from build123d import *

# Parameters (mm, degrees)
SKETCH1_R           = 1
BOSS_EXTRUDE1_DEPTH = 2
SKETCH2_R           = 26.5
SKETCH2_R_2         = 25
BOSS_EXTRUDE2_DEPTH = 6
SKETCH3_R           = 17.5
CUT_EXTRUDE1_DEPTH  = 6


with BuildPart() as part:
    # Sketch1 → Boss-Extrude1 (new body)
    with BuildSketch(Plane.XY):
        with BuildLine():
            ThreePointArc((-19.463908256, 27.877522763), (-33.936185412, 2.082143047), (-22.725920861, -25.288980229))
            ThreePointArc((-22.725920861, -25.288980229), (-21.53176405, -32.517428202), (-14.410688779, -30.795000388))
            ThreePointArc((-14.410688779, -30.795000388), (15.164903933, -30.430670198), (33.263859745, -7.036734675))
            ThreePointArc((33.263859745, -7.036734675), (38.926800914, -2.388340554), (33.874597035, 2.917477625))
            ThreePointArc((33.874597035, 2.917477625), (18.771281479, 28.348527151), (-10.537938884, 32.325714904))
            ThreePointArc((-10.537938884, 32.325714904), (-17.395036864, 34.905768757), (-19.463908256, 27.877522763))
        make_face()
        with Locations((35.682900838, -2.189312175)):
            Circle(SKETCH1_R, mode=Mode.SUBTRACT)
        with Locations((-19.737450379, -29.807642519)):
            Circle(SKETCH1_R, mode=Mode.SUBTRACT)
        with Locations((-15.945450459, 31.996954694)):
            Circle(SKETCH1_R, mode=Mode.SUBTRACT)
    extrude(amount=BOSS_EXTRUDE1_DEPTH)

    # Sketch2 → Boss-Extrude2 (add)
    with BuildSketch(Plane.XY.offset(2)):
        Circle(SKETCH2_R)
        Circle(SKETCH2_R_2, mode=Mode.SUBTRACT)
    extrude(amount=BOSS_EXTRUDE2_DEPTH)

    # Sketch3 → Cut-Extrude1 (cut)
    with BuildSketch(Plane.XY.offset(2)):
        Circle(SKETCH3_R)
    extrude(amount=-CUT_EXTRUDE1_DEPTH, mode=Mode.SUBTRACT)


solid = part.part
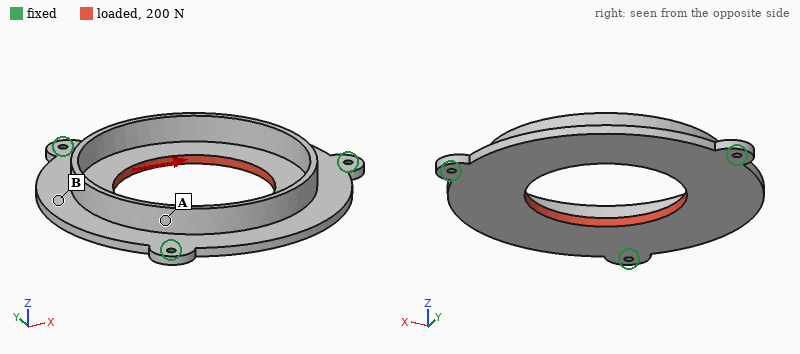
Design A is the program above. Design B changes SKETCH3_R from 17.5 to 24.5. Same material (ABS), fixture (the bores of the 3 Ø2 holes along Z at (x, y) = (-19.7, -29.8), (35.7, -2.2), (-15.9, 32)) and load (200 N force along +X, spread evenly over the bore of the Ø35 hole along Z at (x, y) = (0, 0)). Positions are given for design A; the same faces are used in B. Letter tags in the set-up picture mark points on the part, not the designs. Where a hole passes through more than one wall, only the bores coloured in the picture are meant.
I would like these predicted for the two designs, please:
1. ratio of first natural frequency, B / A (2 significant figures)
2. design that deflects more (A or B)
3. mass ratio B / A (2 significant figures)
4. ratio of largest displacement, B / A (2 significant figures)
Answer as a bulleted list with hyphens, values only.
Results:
- 0.97
- B
- 0.74
- 1.2
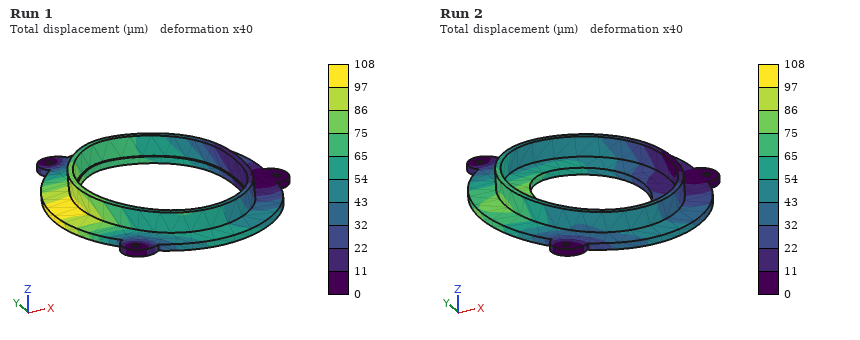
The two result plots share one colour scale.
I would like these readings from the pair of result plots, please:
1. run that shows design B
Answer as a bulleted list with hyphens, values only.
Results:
- Run 1
